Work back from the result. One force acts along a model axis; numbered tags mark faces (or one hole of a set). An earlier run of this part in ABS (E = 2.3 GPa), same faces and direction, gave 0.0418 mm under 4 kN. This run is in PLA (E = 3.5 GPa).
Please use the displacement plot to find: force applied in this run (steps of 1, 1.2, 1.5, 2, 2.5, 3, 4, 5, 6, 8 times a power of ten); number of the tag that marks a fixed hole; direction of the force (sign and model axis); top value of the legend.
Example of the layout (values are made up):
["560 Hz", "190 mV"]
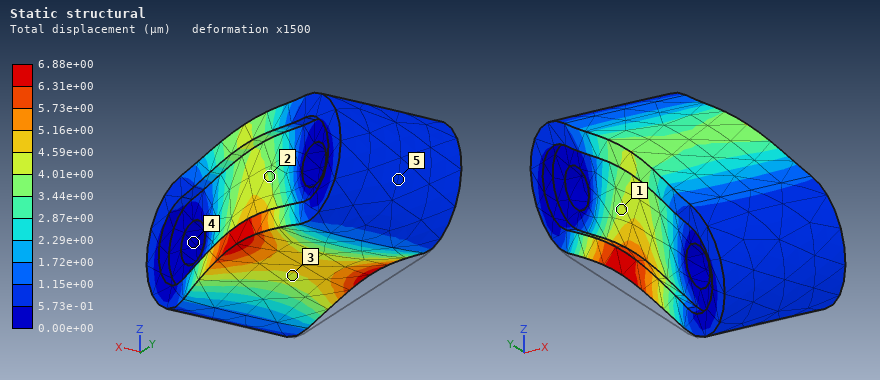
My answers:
["1 kN", "4", "+Z", "6.88e+00 µm"]
